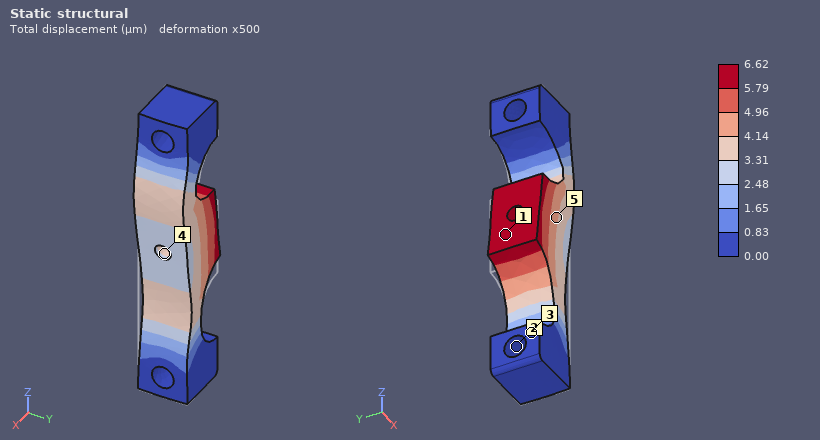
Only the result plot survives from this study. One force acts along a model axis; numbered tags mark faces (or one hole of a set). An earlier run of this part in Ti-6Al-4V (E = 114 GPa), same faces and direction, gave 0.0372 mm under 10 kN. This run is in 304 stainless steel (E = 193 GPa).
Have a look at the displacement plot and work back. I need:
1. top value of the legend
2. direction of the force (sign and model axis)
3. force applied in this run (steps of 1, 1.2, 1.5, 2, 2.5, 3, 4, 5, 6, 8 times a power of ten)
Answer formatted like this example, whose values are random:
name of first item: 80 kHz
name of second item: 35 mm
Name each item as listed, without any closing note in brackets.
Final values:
top value of the legend: 6.62 µm
direction of the force: +Z
force applied in this run: 3 kN
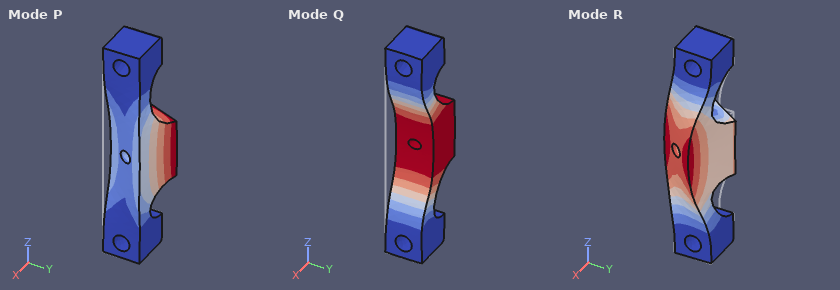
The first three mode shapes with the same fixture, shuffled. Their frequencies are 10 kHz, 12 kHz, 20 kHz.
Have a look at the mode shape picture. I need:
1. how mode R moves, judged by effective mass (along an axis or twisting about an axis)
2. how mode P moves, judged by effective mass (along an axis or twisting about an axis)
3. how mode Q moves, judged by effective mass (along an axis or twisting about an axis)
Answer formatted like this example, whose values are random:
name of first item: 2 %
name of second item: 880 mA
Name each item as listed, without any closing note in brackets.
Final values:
how mode R moves, judged by effective mass: along Y
how mode P moves, judged by effective mass: along Y
how mode Q moves, judged by effective mass: along X
